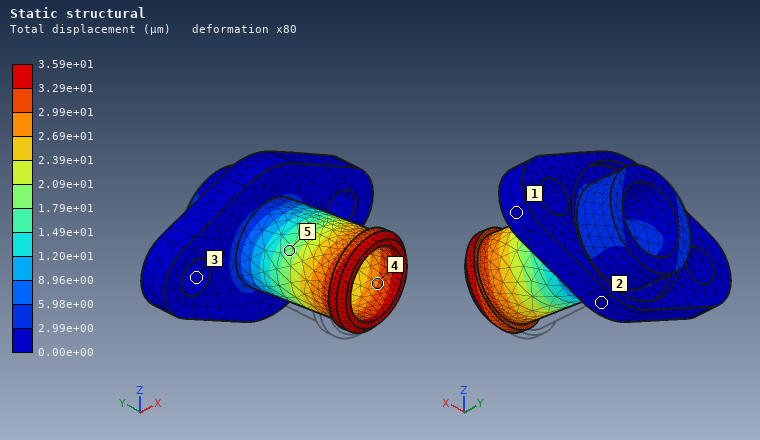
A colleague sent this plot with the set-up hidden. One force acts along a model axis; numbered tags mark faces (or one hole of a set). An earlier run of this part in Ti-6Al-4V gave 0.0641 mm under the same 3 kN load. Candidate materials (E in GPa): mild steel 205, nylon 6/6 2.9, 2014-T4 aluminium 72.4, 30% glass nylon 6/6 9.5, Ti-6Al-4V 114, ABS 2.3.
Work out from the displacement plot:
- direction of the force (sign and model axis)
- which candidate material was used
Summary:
+X
mild steel
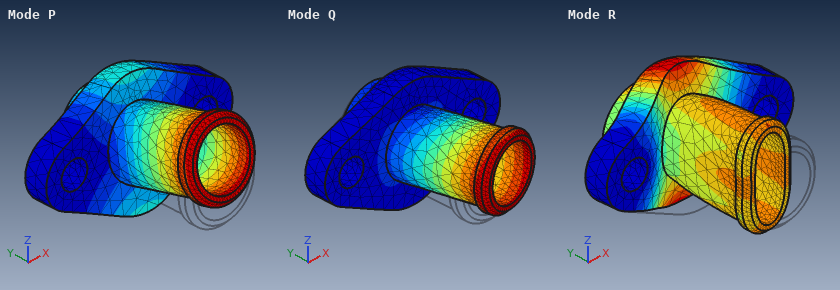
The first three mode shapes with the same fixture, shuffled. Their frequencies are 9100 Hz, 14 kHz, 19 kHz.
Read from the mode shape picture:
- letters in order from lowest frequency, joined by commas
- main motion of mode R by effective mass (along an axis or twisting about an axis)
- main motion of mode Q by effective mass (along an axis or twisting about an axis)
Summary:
P, Q, R
along Y
along X
